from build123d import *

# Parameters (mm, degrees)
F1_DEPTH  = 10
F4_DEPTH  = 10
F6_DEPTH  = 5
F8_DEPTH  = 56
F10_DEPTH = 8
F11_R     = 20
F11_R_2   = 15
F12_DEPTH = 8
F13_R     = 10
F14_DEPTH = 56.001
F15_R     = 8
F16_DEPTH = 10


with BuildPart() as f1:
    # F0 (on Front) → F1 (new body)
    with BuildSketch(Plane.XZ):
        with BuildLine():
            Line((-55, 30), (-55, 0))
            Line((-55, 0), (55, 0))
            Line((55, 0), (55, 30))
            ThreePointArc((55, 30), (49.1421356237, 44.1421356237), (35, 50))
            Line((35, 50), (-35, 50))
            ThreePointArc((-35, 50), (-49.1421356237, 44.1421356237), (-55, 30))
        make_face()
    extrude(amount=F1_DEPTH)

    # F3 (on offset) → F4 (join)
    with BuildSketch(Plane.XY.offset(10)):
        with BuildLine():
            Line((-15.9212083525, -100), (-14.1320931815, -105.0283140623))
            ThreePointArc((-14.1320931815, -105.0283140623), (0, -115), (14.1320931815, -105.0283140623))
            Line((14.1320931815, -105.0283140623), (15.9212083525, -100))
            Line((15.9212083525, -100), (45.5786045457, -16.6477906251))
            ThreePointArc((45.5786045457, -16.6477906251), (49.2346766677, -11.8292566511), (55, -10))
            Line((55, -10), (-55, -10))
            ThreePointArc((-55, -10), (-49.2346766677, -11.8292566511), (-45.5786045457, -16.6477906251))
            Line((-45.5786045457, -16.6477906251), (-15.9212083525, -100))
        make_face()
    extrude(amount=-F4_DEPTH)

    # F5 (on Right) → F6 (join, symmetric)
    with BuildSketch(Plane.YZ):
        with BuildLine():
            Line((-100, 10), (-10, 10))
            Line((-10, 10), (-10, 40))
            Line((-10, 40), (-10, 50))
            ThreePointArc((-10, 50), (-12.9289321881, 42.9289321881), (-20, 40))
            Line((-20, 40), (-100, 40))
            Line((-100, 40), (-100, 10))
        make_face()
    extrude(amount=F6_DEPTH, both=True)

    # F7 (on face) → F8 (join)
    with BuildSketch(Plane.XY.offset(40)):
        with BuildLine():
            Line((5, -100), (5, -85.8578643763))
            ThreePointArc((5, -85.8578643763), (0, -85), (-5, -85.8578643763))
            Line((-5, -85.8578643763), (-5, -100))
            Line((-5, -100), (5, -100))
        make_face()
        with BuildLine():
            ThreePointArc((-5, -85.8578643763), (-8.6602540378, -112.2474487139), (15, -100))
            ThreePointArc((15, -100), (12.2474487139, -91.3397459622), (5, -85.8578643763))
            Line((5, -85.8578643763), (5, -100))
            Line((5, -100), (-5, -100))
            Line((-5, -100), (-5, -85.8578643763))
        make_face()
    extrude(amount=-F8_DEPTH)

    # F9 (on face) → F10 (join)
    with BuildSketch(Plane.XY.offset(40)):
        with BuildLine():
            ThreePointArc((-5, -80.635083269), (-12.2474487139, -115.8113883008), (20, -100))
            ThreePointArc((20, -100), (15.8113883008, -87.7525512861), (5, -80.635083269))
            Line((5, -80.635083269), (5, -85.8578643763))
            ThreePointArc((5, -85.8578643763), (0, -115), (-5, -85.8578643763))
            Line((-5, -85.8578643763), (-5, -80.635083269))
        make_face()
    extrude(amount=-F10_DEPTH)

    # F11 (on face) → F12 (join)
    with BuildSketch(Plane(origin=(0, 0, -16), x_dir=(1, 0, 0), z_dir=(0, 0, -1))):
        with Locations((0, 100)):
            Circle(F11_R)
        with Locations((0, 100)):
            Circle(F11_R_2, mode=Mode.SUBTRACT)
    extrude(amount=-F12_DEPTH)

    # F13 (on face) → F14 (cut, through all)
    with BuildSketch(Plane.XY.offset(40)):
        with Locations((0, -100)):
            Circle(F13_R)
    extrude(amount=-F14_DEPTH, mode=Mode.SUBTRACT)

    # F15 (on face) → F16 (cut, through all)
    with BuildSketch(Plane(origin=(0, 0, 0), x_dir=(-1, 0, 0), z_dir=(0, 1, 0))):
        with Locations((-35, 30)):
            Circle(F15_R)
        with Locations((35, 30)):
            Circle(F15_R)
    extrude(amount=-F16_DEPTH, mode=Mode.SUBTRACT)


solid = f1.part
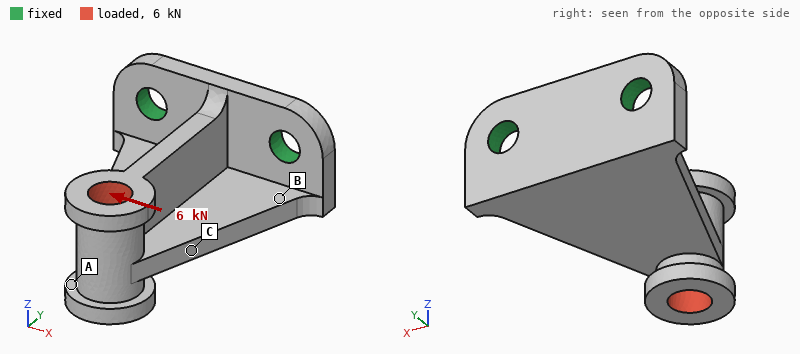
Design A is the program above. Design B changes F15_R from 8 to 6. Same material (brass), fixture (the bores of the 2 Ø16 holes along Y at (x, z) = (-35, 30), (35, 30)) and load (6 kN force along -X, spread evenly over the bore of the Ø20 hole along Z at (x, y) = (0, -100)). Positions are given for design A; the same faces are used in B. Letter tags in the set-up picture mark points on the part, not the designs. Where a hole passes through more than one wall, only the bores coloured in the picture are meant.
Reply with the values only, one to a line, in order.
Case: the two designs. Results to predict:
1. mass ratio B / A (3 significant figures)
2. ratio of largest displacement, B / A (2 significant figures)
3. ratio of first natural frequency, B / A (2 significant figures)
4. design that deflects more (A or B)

1.01
1.1
0.90
B
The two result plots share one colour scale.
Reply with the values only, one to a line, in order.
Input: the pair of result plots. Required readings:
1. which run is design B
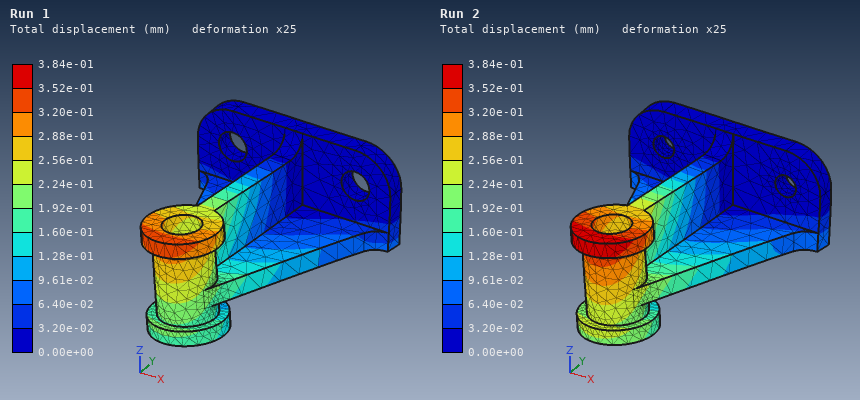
Run 2
